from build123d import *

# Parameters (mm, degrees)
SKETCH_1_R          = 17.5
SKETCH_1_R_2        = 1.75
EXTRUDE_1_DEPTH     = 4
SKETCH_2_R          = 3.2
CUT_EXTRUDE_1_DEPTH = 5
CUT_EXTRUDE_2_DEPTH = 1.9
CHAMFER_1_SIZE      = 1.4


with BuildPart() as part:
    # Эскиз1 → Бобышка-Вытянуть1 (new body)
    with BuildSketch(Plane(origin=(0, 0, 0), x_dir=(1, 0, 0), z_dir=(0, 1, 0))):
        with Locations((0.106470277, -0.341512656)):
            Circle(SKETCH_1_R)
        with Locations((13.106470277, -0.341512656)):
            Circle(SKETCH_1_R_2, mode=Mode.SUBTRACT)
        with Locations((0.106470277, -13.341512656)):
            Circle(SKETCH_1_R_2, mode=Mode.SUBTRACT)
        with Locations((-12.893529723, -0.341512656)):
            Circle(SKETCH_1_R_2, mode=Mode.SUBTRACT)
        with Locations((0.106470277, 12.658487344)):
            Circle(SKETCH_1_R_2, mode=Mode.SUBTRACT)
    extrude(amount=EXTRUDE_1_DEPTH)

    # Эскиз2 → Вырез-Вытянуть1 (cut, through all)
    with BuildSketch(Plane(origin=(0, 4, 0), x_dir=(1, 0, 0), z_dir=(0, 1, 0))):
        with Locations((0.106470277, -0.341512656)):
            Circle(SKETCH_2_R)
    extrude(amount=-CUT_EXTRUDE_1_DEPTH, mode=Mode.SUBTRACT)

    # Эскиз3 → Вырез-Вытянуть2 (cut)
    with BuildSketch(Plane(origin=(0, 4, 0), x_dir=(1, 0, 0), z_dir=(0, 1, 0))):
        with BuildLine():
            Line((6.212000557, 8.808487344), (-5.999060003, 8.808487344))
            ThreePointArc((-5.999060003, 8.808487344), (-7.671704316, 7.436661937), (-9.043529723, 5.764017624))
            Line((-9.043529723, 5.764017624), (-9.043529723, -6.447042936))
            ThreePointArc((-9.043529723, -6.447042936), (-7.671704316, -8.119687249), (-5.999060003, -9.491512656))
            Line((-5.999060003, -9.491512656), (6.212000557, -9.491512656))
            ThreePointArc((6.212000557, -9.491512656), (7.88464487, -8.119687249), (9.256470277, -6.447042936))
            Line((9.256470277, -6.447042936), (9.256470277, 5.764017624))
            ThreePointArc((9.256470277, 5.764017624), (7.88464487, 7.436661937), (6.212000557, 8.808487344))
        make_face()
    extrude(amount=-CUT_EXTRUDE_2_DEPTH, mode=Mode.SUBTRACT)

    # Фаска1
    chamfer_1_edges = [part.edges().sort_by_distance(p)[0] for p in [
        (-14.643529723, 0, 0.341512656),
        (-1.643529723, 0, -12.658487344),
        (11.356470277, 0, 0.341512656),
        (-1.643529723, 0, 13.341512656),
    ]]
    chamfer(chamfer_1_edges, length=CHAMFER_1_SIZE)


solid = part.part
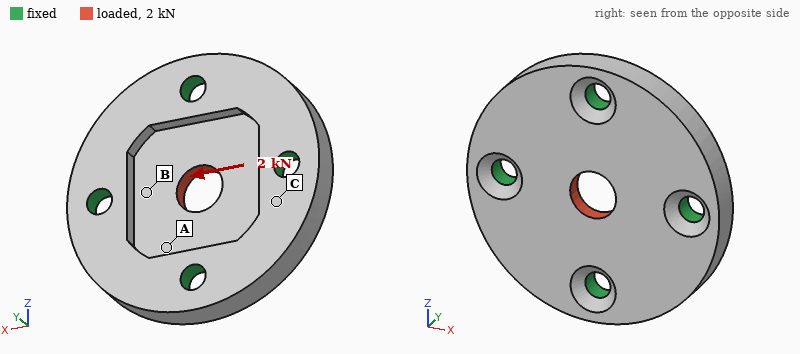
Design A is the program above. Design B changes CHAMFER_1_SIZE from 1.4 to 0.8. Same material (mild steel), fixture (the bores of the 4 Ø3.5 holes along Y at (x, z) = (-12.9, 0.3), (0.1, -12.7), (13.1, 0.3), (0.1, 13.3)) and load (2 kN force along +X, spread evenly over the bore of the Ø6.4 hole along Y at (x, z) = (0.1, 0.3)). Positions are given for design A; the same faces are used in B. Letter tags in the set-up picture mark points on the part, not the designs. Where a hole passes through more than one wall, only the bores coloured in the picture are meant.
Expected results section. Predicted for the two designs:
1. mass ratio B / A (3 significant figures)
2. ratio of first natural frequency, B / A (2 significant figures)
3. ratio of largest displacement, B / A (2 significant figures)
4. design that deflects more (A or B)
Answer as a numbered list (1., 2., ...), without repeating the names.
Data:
1. 1.01
2. 1.1
3. 0.92
4. A
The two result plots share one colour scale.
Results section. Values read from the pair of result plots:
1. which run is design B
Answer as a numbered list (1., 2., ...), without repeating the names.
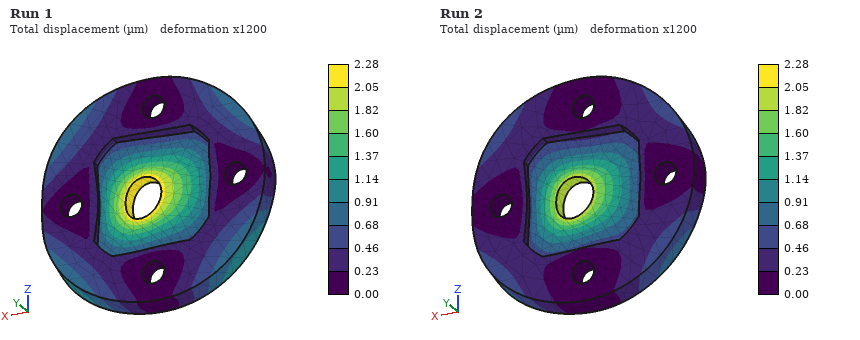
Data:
1. Run 2
